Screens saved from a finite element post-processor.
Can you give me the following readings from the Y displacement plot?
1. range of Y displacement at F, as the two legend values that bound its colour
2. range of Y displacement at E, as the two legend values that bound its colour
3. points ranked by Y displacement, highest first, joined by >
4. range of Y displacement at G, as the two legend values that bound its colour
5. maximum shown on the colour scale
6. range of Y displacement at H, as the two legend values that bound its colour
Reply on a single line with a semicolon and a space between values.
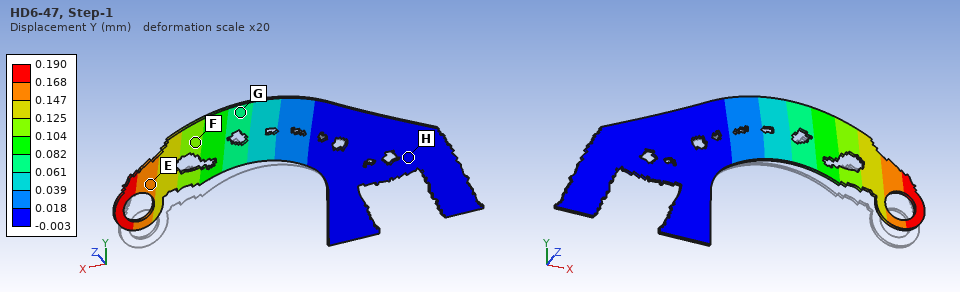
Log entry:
0.104 to 0.125 mm; 0.147 to 0.168 mm; E > F > G > H; 0.061 to 0.082 mm; 0.190 mm; -0.003 to 0.018 mm
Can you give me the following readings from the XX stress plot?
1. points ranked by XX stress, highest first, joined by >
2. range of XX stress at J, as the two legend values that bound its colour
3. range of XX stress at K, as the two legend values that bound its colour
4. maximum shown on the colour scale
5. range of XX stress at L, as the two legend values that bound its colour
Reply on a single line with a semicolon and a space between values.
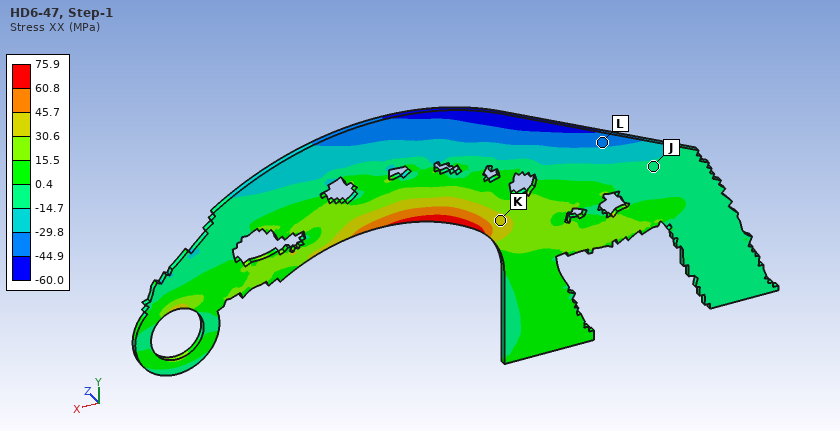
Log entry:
K > J > L; -14.7 to 0.4 MPa; 30.6 to 45.7 MPa; 75.9 MPa; -44.9 to -29.8 MPa
